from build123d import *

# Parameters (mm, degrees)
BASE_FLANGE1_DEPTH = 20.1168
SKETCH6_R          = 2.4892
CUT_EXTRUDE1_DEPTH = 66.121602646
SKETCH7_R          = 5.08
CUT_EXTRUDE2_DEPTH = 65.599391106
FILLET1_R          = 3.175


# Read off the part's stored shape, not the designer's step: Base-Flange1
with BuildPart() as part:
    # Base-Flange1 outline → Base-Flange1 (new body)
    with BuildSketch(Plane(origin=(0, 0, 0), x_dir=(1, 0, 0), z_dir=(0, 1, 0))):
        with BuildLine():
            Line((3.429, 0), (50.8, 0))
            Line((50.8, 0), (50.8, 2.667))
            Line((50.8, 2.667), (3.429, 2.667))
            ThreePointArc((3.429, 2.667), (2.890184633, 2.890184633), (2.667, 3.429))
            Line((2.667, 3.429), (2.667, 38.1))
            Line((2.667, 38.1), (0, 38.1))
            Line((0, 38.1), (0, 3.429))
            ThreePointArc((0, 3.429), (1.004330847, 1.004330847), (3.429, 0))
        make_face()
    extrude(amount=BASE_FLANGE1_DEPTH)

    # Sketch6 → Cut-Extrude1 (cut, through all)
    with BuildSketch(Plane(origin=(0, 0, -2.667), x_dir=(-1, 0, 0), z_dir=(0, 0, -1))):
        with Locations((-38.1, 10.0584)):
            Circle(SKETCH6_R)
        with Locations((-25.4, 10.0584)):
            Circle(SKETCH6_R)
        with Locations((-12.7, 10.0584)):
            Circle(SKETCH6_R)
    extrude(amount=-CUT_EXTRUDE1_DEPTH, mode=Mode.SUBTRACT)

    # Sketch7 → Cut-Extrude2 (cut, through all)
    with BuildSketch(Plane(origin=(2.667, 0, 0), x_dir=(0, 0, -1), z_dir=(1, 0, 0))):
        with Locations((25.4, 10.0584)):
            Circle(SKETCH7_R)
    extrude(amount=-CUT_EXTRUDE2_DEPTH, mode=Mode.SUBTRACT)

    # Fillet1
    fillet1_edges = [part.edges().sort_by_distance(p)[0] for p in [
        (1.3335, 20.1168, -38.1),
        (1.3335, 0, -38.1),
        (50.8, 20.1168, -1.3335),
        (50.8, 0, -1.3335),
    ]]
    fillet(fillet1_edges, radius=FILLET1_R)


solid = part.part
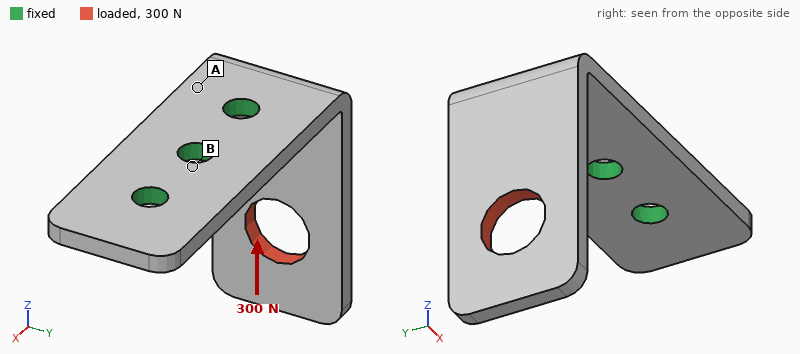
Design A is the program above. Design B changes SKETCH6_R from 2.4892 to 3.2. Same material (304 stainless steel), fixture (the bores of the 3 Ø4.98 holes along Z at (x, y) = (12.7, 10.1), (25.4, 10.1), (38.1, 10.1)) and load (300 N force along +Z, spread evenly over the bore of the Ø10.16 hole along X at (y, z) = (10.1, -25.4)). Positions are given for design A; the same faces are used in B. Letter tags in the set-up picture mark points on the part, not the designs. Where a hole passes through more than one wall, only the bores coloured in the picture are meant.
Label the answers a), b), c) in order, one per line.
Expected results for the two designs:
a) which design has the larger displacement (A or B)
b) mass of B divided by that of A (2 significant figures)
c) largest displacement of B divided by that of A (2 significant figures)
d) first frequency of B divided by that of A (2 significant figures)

a) A
b) 0.98
c) 0.84
d) 1.0
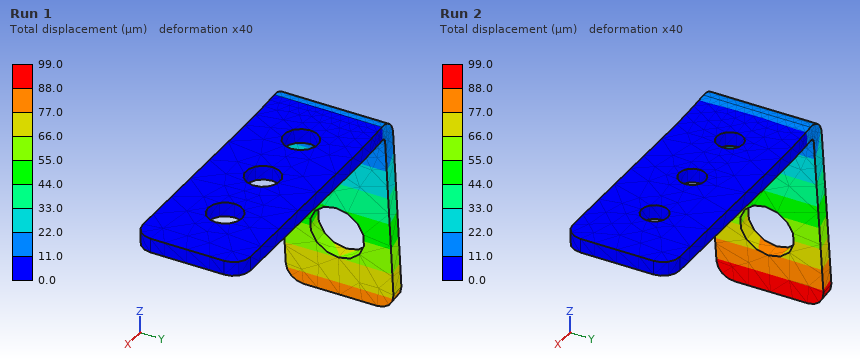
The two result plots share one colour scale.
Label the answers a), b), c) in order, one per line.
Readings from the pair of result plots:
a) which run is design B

a) Run 1
